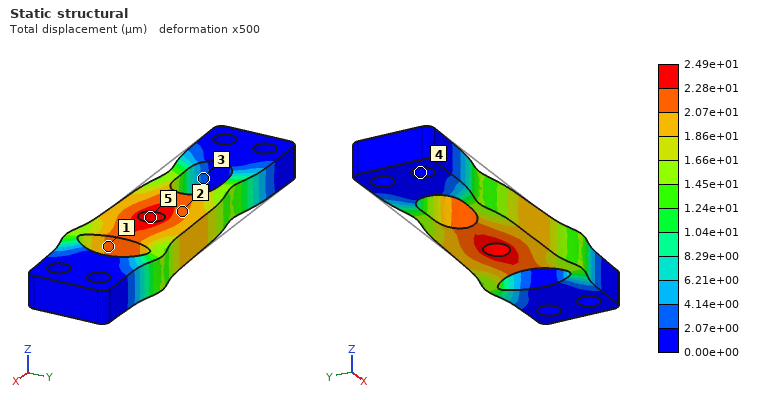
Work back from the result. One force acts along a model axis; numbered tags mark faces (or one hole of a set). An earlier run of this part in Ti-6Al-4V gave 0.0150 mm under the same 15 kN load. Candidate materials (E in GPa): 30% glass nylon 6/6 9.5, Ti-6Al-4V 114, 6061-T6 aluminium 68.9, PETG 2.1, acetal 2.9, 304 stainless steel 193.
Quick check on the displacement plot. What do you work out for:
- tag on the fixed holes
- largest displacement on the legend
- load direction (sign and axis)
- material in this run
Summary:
4
2.49e+01 µm
+X
6061-T6 aluminium
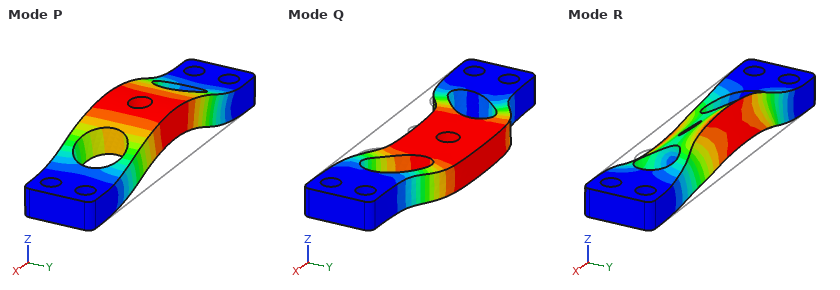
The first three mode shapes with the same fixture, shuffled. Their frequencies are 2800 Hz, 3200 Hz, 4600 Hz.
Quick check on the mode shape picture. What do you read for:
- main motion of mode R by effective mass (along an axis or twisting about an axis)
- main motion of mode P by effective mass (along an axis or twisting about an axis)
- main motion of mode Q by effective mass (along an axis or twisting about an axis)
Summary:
twisting about X
along Z
along Y
